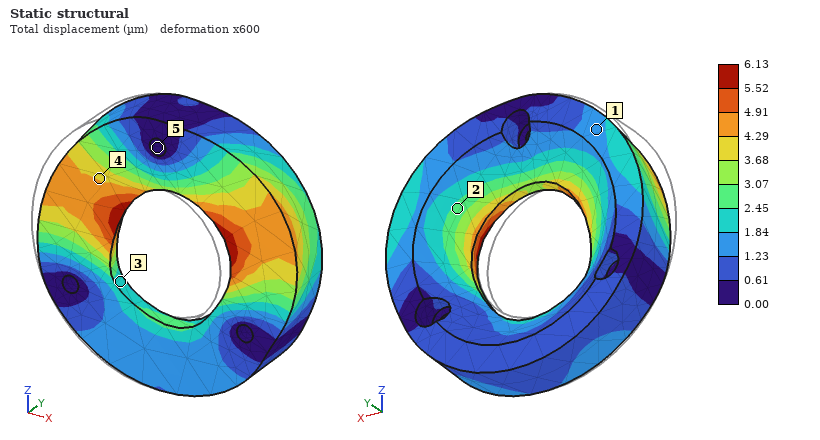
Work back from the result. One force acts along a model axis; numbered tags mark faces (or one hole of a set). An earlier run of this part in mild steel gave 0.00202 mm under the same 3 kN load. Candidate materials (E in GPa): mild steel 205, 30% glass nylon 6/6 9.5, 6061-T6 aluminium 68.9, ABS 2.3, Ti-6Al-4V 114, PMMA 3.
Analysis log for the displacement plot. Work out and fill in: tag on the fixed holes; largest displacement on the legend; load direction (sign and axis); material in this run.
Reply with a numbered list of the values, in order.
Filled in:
1. 5
2. 6.13 µm
3. +X
4. 6061-T6 aluminium
